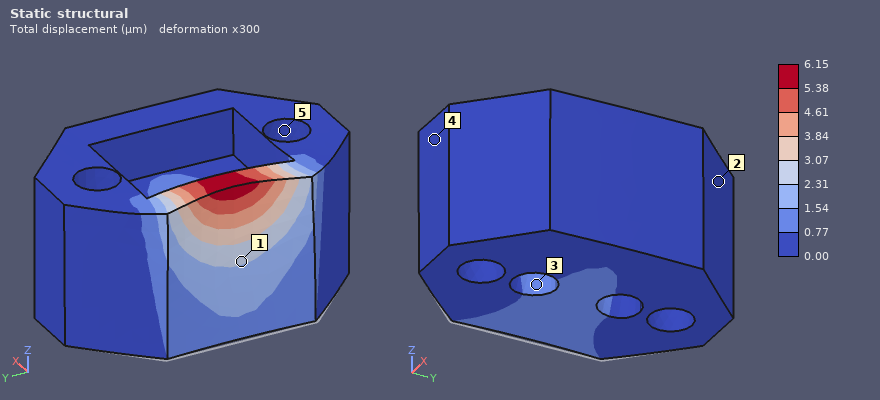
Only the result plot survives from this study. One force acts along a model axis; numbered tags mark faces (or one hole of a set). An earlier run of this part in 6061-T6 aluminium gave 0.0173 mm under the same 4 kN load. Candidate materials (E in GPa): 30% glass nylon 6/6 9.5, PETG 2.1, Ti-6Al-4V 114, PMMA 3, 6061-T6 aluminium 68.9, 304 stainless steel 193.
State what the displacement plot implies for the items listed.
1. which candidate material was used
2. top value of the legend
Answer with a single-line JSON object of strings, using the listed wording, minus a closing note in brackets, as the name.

{"which candidate material was used": "304 stainless steel", "top value of the legend": "6.15 µm"}
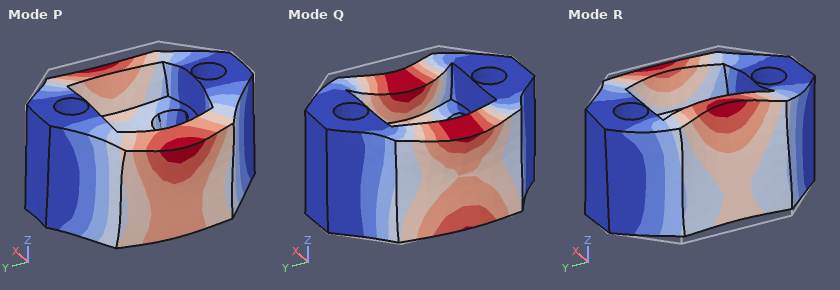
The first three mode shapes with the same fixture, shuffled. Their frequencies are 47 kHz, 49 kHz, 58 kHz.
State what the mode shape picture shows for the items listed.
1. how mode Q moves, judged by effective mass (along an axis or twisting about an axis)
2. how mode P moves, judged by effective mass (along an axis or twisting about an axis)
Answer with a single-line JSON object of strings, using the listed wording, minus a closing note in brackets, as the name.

{"how mode Q moves, judged by effective mass": "along X", "how mode P moves, judged by effective mass": "along Z"}
